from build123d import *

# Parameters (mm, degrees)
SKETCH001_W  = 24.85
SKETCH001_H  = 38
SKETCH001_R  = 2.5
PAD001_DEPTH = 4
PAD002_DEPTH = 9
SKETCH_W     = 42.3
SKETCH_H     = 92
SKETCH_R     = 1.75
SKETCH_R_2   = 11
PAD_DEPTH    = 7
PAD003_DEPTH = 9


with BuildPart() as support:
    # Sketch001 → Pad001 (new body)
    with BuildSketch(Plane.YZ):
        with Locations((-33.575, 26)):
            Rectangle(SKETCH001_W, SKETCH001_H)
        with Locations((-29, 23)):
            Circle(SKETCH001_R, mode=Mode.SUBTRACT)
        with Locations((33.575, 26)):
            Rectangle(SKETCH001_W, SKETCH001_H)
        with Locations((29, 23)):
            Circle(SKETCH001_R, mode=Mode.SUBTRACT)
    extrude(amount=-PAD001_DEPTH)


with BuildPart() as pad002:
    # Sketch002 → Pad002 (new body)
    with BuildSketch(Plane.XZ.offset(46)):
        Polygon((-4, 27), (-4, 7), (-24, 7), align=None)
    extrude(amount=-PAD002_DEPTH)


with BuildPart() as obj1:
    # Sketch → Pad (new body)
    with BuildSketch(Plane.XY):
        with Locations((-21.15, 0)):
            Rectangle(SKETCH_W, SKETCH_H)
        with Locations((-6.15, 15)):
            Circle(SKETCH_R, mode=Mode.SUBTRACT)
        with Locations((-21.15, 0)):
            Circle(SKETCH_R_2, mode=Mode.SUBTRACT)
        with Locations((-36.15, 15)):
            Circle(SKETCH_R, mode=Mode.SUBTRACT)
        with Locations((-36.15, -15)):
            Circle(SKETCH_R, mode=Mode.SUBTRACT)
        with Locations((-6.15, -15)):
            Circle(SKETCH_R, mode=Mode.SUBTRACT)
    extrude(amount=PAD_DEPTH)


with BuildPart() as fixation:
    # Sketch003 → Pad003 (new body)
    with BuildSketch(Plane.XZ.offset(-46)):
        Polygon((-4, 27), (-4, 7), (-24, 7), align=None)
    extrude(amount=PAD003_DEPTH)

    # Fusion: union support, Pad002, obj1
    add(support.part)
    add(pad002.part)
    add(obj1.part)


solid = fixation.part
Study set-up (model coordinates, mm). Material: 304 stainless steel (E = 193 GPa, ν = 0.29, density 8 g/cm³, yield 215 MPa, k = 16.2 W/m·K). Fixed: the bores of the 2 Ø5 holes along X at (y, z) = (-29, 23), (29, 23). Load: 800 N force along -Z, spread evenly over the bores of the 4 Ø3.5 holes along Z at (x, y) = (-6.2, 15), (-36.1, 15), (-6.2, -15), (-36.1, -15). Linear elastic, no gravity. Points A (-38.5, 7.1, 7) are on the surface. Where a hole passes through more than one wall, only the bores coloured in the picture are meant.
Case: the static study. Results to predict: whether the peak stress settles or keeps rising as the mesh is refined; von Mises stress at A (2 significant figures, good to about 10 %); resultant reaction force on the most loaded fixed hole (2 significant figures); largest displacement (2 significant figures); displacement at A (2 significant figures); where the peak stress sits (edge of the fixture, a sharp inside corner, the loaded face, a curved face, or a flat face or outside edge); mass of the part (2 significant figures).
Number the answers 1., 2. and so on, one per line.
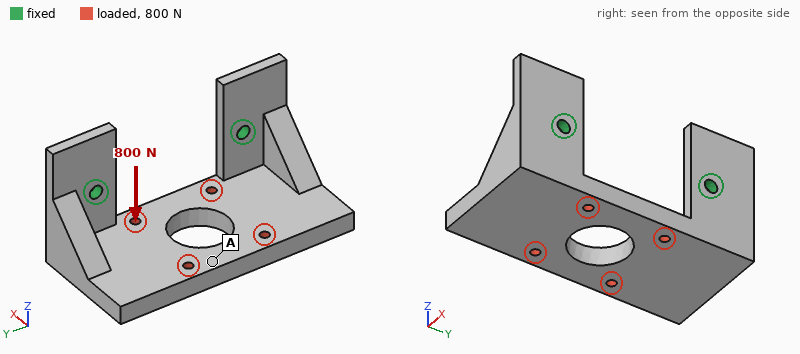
1. keeps rising
2. 15 MPa
3. 440 N
4. 95 µm
5. 82 µm
6. edge of the fixture
7. 280 g
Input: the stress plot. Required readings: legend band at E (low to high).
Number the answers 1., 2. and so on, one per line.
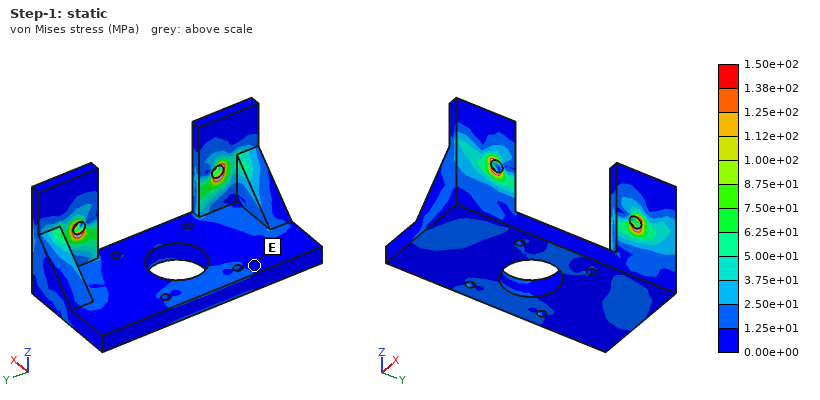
1. 0.00e+00 to 1.25e+01 MPa
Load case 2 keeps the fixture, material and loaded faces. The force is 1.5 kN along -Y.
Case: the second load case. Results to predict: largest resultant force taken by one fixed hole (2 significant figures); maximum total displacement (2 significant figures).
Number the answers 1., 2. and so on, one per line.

1. 880 N
2. 32 µm
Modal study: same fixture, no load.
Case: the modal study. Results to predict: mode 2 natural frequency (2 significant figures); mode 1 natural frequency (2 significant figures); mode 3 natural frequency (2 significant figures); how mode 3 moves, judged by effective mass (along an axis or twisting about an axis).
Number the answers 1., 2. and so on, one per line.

1. 2100 Hz
2. 1200 Hz
3. 3700 Hz
4. along Y
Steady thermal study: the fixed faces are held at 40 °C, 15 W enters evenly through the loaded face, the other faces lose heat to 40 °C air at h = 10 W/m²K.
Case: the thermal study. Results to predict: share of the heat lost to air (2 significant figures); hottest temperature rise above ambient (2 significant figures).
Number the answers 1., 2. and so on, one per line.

1. 42 %
2. 83 K
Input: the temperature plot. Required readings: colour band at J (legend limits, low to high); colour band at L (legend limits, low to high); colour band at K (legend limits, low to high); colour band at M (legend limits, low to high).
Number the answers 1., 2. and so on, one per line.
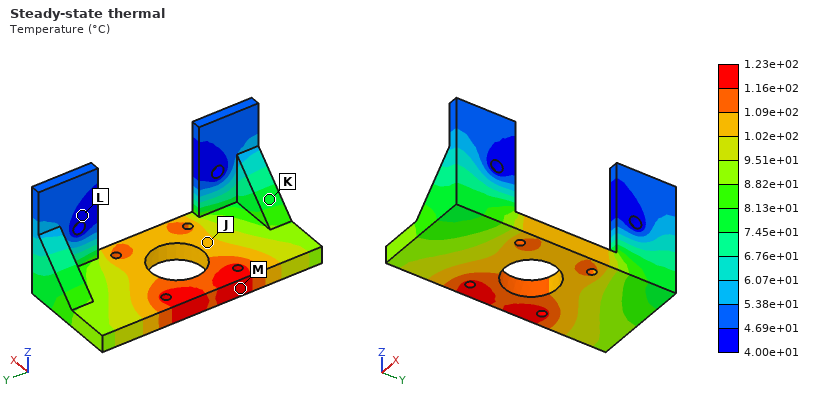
1. 1.02e+02 to 1.09e+02 °C
2. 4.00e+01 to 4.69e+01 °C
3. 7.45e+01 to 8.13e+01 °C
4. 1.16e+02 to 1.23e+02 °C
